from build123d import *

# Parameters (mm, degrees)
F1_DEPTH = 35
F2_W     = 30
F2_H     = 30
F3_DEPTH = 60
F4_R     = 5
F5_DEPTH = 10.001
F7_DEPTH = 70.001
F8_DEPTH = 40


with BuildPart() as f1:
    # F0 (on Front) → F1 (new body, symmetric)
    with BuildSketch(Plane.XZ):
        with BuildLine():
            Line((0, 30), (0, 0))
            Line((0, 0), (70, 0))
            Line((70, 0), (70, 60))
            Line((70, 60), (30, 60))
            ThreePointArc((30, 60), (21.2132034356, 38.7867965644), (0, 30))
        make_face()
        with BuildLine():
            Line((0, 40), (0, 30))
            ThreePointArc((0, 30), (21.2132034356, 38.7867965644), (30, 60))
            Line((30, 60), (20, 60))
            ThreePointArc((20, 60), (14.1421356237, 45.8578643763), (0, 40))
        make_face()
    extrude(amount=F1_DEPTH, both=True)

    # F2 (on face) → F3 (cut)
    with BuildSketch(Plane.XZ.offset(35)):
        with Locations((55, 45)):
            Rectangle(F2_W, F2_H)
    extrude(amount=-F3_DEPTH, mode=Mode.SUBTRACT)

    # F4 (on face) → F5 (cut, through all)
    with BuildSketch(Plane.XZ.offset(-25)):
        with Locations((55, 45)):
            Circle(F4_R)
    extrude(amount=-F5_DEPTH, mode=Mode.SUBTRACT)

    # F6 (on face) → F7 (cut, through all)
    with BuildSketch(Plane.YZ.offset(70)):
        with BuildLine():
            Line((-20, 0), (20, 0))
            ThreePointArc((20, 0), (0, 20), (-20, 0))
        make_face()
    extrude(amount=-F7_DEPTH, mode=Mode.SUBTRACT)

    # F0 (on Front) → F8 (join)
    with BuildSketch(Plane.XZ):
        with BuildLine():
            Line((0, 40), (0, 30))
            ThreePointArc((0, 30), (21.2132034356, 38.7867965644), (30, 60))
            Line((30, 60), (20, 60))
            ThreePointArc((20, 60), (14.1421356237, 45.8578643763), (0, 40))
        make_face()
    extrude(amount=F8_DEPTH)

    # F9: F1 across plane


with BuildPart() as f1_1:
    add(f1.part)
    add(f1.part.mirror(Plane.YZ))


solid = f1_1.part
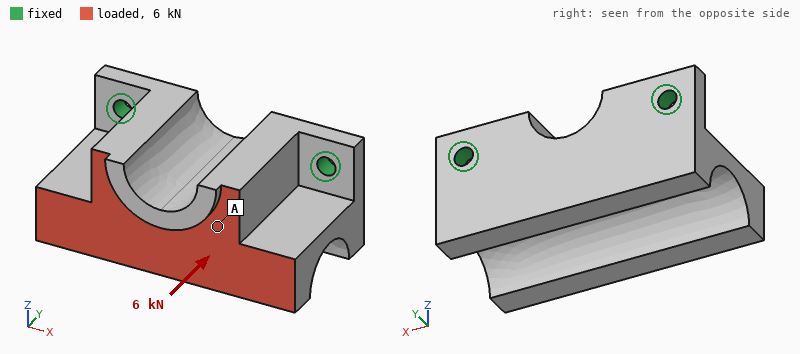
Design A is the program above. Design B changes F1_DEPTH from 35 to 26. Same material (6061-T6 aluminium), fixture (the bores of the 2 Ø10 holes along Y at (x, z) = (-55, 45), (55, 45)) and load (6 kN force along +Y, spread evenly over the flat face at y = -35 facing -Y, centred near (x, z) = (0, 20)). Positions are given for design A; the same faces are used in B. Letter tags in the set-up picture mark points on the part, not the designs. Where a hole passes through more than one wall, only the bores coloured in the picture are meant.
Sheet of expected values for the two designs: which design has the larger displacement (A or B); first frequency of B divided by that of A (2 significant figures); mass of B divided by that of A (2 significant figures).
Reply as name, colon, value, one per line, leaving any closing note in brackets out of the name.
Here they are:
which design has the larger displacement: B
first frequency of B divided by that of A: 0.092
mass of B divided by that of A: 0.67
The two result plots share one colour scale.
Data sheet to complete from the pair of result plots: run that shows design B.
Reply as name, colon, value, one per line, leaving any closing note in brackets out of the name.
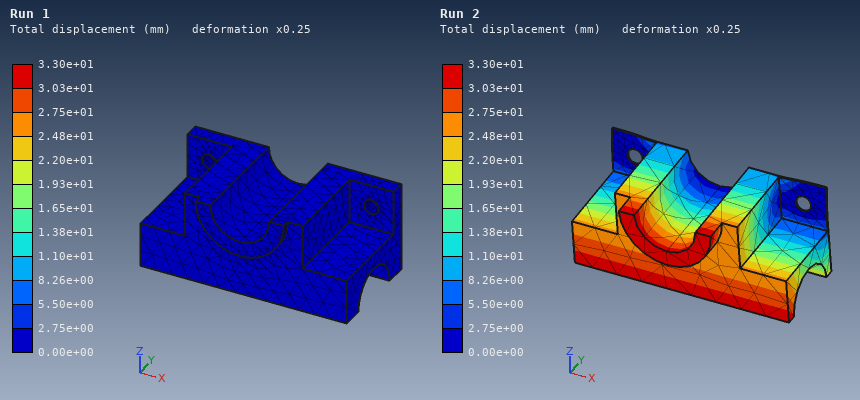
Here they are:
run that shows design B: Run 2
